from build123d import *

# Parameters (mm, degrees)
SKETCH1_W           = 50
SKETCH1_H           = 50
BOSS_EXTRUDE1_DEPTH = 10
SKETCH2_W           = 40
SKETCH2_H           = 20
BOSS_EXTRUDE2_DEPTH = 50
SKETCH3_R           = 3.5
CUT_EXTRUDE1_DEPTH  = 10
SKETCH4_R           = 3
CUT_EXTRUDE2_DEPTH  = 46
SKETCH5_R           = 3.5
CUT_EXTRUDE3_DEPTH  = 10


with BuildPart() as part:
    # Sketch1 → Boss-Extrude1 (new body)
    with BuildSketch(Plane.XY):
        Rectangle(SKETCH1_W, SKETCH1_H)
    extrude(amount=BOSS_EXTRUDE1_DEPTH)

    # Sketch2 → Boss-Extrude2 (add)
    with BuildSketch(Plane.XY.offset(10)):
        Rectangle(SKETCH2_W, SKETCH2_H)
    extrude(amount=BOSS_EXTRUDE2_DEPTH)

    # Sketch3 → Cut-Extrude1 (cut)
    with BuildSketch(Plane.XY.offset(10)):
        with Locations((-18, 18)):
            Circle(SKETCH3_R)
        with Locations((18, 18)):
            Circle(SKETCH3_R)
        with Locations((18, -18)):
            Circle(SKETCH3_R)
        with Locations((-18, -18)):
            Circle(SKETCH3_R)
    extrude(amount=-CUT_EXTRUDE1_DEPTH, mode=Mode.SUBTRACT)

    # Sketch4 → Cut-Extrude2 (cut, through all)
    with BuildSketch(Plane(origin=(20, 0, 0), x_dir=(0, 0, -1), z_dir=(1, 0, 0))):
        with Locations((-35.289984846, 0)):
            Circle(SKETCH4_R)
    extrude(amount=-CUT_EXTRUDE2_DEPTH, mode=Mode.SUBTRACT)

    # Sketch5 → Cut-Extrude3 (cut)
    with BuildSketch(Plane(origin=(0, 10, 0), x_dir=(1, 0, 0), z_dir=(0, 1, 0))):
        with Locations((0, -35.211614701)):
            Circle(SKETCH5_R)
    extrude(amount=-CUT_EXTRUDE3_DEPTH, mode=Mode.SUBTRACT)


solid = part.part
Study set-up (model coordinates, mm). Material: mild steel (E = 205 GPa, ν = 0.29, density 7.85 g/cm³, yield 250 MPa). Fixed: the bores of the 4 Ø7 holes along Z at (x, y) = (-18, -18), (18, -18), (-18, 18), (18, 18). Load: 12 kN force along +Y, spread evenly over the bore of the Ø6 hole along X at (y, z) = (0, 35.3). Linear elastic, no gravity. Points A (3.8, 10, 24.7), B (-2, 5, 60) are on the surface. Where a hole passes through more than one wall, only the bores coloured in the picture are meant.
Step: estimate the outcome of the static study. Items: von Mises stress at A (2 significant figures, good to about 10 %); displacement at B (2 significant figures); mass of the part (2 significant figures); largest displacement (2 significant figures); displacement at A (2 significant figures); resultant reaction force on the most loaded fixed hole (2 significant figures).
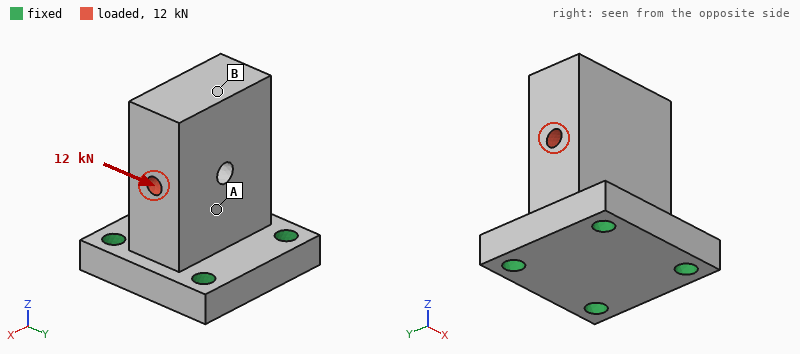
43 MPa
66 µm
490 g
67 µm
22 µm
6.9 kN
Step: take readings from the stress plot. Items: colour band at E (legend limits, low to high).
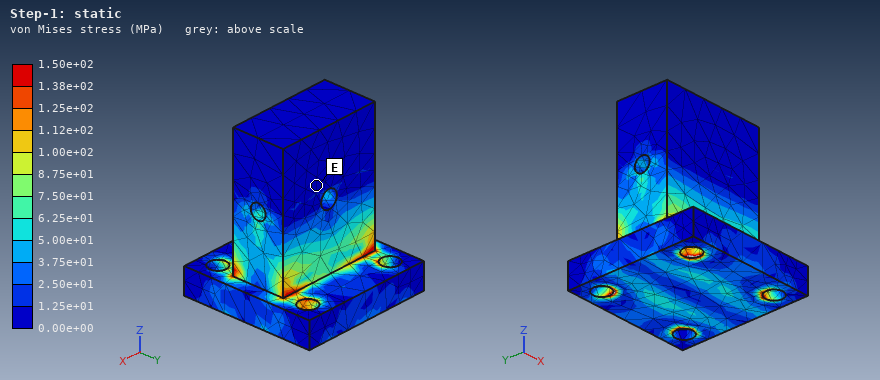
0.00e+00 to 1.25e+01 MPa
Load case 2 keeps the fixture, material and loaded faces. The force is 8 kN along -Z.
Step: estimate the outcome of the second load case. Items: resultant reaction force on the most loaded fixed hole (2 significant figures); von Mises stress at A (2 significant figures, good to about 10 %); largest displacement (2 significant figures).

2.1 kN
6.3 MPa
3.9 µm
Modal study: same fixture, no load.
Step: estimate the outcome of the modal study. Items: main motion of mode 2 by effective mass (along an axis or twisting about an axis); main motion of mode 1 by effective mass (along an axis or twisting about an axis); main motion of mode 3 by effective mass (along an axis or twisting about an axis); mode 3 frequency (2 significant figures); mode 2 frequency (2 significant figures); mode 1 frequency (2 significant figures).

along X
along Y
twisting about Z
11 kHz
6200 Hz
4500 Hz
